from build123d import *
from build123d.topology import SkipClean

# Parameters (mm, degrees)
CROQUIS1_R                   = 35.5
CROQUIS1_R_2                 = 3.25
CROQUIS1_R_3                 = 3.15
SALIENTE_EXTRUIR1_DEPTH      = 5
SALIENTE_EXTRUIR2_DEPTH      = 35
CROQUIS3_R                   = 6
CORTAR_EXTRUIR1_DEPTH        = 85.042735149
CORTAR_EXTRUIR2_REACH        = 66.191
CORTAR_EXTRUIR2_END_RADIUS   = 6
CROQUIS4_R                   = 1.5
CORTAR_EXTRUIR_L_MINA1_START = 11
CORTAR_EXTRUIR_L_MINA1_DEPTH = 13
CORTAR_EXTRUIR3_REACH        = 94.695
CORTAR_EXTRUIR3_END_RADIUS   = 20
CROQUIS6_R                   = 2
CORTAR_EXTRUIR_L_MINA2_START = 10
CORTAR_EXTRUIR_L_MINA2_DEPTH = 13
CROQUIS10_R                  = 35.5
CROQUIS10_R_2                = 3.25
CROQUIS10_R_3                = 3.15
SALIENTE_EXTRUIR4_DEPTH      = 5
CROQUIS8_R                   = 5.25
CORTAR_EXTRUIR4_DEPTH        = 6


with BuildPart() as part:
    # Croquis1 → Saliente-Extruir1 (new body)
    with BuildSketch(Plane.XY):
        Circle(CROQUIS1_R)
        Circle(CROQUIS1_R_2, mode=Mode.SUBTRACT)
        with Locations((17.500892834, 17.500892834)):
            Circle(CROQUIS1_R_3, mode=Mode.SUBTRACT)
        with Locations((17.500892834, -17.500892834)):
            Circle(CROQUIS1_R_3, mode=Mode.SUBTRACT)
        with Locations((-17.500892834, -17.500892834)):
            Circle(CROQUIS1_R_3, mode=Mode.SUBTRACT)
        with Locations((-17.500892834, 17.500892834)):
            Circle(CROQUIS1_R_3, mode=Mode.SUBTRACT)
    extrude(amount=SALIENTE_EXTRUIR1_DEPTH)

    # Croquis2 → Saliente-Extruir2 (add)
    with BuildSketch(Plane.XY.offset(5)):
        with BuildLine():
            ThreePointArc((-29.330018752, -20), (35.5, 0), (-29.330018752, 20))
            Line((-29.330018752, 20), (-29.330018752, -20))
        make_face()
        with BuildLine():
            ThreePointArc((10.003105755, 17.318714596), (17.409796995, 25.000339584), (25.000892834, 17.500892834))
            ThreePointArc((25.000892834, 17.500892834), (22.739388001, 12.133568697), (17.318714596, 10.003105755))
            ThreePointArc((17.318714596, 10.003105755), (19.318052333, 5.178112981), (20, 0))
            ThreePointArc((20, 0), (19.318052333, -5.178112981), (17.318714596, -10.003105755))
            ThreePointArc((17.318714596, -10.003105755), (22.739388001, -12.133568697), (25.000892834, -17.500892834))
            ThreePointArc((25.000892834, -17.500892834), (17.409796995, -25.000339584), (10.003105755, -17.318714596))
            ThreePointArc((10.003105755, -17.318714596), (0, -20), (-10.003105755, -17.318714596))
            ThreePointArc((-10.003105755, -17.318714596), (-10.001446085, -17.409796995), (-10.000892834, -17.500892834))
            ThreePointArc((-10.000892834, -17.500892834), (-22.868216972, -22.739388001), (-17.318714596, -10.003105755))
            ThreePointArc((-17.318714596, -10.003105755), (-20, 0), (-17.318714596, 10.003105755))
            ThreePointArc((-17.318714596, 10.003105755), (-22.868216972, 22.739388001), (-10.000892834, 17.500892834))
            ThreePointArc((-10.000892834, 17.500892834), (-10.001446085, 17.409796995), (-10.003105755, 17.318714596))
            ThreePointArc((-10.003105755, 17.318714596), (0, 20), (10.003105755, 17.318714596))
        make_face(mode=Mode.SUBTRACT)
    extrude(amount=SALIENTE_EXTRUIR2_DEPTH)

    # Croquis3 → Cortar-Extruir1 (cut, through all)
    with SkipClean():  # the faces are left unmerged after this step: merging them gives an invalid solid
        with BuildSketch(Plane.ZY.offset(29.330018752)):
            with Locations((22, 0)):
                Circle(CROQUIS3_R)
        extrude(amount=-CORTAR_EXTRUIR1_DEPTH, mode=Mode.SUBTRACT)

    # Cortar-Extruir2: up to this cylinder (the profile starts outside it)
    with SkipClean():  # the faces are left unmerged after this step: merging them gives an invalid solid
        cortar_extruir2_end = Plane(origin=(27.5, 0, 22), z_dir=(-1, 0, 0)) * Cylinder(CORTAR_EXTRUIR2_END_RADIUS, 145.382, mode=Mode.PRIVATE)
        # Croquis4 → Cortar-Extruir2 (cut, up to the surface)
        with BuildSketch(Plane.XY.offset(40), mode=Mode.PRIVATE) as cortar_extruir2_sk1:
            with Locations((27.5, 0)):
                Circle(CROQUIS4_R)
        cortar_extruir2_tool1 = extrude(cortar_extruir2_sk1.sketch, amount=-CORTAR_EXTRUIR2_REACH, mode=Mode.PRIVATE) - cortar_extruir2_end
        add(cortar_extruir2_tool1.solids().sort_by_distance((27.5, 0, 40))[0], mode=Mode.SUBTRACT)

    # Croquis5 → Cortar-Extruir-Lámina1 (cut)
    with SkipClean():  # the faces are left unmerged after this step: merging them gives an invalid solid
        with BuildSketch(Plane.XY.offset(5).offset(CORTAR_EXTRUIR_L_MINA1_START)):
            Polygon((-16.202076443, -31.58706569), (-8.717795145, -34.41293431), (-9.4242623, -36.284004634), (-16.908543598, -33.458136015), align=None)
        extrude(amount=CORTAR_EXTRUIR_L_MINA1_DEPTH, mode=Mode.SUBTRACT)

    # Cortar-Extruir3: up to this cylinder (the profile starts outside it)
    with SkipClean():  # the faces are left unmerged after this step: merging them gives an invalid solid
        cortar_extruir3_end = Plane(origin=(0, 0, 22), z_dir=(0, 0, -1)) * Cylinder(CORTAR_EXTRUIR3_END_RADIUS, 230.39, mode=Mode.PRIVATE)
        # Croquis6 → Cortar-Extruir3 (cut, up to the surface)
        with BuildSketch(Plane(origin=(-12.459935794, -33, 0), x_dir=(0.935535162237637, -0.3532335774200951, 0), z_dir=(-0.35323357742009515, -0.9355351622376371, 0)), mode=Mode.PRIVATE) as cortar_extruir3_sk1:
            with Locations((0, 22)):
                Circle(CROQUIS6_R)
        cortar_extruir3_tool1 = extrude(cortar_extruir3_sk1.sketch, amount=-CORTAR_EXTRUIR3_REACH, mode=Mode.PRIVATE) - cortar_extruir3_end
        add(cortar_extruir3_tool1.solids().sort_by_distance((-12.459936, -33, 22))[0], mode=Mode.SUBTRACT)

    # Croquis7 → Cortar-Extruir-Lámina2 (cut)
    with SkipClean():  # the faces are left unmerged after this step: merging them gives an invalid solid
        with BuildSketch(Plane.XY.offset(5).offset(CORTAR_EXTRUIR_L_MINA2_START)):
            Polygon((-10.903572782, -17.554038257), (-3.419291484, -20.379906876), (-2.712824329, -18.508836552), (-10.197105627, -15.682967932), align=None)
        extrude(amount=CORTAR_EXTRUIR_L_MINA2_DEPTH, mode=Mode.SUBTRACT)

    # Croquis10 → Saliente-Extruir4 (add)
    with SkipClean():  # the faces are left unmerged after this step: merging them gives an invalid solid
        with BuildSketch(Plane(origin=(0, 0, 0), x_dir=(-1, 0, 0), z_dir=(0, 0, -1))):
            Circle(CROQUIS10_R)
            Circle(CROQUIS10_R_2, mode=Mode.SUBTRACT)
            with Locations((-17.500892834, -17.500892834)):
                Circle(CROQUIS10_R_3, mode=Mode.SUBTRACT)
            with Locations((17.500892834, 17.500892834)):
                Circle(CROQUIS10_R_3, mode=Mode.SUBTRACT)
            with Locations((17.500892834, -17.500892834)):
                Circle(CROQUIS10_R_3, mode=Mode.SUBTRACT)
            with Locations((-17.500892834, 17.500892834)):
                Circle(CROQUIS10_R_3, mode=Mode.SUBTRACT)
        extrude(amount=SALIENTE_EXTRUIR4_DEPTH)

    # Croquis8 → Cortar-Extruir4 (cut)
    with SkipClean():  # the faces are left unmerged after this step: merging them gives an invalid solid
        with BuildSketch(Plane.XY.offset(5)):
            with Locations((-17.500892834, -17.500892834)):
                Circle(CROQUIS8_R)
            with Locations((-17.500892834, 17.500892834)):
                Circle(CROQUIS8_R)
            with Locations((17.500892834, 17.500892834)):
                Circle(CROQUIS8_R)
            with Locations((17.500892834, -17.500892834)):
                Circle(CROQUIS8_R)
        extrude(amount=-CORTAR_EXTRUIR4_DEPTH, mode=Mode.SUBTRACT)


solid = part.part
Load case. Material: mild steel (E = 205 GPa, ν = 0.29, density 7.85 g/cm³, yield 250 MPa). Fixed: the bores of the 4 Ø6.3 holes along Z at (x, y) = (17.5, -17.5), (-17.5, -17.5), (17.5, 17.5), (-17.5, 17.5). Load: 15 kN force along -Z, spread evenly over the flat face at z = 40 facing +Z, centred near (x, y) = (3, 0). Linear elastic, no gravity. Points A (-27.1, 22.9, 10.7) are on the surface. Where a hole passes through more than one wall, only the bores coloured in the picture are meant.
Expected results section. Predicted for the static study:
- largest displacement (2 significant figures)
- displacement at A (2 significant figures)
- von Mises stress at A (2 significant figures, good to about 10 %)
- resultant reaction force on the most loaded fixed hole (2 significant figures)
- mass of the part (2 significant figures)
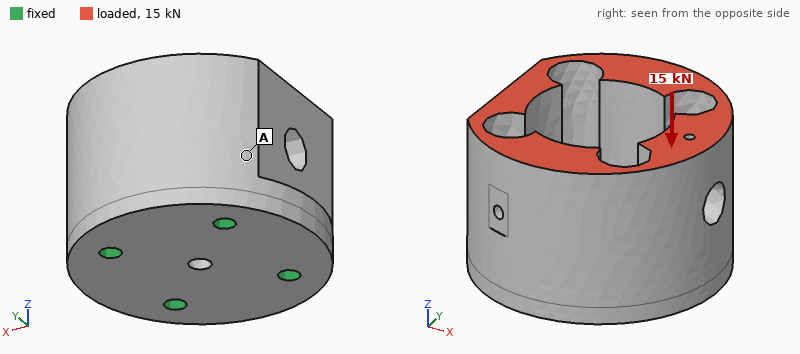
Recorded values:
6.4 µm
2.7 µm
12 MPa
4.3 kN
790 g
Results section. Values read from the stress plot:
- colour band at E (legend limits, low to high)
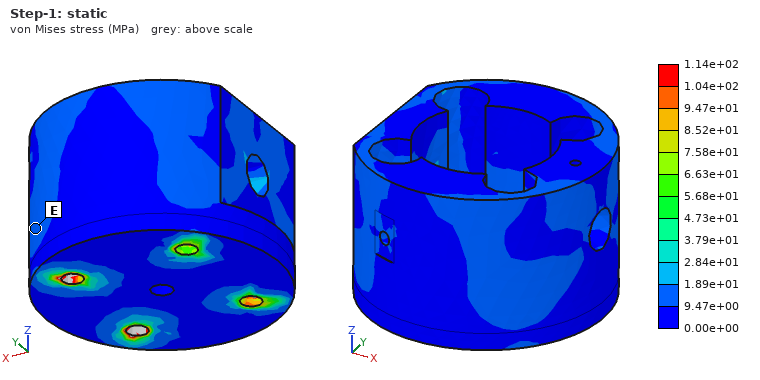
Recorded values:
9.47e+00 to 1.89e+01 MPa
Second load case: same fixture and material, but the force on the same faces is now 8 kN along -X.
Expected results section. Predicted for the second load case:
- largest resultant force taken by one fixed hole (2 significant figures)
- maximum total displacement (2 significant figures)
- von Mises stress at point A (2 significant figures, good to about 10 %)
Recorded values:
5.1 kN
37 µm
22 MPa
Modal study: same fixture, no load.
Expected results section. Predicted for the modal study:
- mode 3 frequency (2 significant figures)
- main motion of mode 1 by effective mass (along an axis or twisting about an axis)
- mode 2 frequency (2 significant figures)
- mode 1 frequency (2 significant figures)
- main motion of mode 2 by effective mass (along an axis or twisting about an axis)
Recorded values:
6800 Hz
along Y
6100 Hz
5600 Hz
along X
